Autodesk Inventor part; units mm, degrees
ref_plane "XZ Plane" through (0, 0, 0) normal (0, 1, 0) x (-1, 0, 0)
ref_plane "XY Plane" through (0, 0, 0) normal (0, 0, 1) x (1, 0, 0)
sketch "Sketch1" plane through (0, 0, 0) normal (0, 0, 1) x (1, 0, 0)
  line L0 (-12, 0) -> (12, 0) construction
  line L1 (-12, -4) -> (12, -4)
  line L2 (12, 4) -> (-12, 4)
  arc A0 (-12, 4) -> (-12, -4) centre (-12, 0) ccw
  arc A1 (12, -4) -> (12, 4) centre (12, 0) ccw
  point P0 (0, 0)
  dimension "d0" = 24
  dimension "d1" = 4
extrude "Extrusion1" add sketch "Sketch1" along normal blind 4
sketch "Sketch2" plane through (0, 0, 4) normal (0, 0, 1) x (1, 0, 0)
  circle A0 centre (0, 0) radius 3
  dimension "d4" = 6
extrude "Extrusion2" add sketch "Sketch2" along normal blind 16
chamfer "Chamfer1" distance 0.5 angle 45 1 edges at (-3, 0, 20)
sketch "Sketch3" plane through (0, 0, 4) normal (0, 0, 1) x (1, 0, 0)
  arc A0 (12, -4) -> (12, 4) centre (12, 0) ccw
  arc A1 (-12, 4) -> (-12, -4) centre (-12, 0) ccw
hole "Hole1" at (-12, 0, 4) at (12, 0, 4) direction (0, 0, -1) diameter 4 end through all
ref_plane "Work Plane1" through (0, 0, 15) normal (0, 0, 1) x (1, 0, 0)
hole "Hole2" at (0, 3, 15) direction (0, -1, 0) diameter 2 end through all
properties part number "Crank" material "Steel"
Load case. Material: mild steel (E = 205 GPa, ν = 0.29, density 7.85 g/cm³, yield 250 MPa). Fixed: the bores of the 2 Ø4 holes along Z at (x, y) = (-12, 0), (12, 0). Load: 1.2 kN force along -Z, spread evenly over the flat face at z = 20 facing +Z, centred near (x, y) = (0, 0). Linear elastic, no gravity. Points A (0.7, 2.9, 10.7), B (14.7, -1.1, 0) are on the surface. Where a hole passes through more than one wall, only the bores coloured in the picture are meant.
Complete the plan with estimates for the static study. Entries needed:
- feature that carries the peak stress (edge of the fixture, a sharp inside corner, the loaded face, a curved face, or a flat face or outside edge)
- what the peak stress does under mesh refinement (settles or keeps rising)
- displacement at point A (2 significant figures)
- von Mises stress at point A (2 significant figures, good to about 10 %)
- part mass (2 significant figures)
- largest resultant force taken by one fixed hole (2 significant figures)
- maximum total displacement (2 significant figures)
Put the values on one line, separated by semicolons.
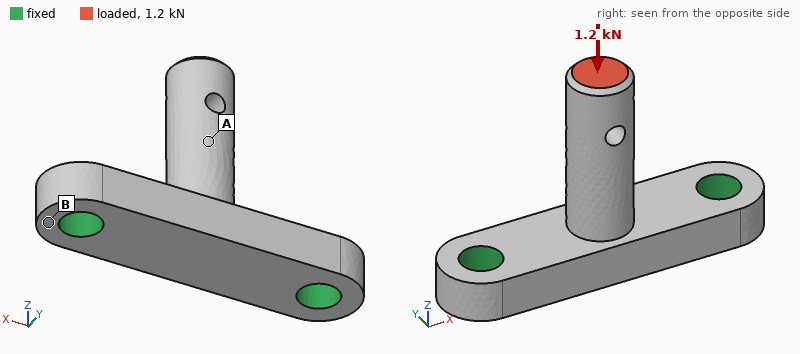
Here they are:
edge of the fixture; keeps rising; 8.9 µm; 38 MPa; 10 g; 610 N; 12 µm
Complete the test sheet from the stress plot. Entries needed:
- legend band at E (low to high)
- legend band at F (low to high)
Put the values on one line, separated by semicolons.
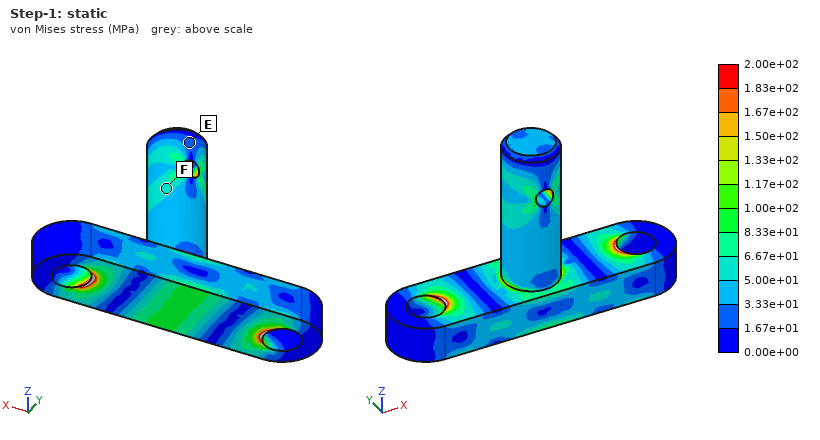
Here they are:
1.67e+01 to 3.33e+01 MPa; 5.00e+01 to 6.67e+01 MPa
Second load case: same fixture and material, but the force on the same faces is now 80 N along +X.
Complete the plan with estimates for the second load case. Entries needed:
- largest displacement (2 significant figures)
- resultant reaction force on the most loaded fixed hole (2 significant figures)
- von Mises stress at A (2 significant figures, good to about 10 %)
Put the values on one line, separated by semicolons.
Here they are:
14 µm; 100 N; 9.9 MPa
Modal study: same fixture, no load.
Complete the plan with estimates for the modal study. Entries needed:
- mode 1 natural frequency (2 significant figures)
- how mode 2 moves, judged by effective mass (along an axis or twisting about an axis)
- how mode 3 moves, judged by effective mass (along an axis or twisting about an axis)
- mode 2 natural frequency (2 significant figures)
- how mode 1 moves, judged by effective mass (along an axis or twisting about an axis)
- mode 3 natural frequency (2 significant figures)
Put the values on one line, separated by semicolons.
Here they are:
9000 Hz; along X; along Z; 12 kHz; along Y; 25 kHz
